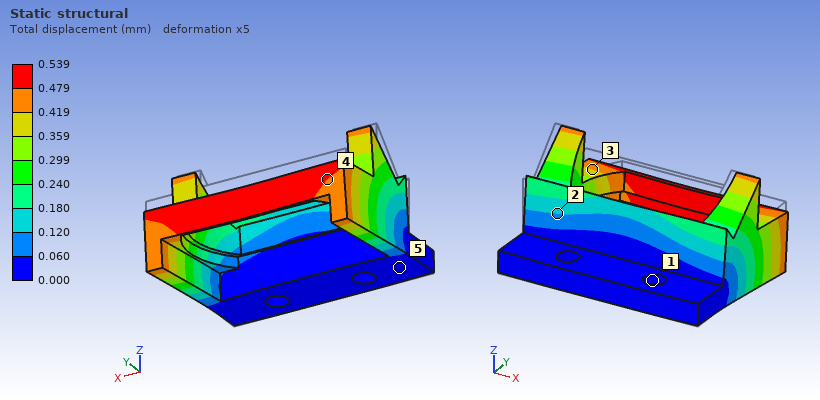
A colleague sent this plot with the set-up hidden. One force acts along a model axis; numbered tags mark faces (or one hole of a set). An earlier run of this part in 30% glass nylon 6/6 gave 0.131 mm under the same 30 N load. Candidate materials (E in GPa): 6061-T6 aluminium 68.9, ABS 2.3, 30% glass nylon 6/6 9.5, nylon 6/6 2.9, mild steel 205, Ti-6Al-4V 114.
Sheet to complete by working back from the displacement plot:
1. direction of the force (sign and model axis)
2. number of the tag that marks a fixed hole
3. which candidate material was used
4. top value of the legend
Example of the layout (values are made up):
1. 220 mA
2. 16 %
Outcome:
1. -Z
2. 1
3. ABS
4. 0.539 mm
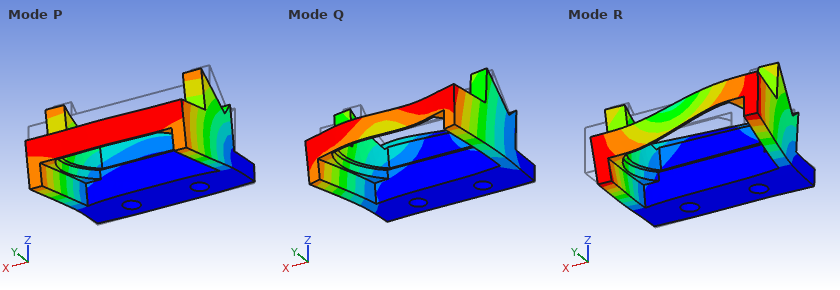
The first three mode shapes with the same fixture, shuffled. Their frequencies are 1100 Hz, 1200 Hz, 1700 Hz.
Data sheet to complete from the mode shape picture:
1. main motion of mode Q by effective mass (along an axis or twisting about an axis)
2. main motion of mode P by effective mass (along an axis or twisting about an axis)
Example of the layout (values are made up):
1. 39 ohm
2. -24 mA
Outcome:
1. along X
2. along Z
